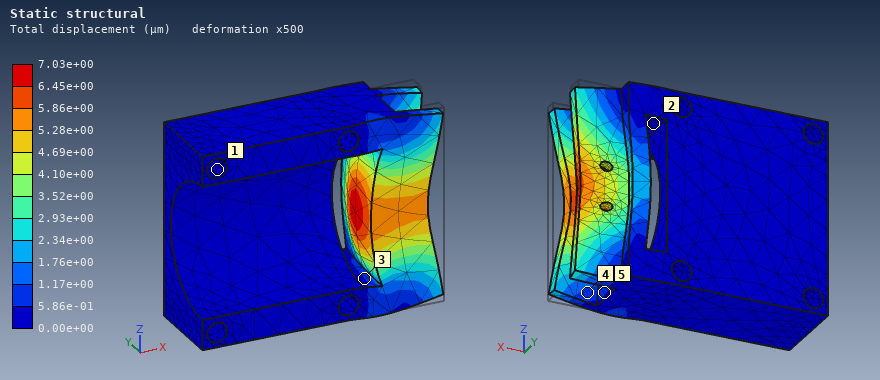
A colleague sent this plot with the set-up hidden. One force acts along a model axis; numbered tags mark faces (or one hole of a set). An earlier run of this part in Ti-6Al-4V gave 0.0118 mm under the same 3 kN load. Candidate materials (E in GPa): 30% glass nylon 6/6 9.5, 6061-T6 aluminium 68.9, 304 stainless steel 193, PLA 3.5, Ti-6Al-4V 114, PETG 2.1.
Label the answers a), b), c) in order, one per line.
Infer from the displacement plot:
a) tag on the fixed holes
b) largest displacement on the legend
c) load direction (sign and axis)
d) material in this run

a) 1
b) 7.03e+00 µm
c) -X
d) 304 stainless steel
